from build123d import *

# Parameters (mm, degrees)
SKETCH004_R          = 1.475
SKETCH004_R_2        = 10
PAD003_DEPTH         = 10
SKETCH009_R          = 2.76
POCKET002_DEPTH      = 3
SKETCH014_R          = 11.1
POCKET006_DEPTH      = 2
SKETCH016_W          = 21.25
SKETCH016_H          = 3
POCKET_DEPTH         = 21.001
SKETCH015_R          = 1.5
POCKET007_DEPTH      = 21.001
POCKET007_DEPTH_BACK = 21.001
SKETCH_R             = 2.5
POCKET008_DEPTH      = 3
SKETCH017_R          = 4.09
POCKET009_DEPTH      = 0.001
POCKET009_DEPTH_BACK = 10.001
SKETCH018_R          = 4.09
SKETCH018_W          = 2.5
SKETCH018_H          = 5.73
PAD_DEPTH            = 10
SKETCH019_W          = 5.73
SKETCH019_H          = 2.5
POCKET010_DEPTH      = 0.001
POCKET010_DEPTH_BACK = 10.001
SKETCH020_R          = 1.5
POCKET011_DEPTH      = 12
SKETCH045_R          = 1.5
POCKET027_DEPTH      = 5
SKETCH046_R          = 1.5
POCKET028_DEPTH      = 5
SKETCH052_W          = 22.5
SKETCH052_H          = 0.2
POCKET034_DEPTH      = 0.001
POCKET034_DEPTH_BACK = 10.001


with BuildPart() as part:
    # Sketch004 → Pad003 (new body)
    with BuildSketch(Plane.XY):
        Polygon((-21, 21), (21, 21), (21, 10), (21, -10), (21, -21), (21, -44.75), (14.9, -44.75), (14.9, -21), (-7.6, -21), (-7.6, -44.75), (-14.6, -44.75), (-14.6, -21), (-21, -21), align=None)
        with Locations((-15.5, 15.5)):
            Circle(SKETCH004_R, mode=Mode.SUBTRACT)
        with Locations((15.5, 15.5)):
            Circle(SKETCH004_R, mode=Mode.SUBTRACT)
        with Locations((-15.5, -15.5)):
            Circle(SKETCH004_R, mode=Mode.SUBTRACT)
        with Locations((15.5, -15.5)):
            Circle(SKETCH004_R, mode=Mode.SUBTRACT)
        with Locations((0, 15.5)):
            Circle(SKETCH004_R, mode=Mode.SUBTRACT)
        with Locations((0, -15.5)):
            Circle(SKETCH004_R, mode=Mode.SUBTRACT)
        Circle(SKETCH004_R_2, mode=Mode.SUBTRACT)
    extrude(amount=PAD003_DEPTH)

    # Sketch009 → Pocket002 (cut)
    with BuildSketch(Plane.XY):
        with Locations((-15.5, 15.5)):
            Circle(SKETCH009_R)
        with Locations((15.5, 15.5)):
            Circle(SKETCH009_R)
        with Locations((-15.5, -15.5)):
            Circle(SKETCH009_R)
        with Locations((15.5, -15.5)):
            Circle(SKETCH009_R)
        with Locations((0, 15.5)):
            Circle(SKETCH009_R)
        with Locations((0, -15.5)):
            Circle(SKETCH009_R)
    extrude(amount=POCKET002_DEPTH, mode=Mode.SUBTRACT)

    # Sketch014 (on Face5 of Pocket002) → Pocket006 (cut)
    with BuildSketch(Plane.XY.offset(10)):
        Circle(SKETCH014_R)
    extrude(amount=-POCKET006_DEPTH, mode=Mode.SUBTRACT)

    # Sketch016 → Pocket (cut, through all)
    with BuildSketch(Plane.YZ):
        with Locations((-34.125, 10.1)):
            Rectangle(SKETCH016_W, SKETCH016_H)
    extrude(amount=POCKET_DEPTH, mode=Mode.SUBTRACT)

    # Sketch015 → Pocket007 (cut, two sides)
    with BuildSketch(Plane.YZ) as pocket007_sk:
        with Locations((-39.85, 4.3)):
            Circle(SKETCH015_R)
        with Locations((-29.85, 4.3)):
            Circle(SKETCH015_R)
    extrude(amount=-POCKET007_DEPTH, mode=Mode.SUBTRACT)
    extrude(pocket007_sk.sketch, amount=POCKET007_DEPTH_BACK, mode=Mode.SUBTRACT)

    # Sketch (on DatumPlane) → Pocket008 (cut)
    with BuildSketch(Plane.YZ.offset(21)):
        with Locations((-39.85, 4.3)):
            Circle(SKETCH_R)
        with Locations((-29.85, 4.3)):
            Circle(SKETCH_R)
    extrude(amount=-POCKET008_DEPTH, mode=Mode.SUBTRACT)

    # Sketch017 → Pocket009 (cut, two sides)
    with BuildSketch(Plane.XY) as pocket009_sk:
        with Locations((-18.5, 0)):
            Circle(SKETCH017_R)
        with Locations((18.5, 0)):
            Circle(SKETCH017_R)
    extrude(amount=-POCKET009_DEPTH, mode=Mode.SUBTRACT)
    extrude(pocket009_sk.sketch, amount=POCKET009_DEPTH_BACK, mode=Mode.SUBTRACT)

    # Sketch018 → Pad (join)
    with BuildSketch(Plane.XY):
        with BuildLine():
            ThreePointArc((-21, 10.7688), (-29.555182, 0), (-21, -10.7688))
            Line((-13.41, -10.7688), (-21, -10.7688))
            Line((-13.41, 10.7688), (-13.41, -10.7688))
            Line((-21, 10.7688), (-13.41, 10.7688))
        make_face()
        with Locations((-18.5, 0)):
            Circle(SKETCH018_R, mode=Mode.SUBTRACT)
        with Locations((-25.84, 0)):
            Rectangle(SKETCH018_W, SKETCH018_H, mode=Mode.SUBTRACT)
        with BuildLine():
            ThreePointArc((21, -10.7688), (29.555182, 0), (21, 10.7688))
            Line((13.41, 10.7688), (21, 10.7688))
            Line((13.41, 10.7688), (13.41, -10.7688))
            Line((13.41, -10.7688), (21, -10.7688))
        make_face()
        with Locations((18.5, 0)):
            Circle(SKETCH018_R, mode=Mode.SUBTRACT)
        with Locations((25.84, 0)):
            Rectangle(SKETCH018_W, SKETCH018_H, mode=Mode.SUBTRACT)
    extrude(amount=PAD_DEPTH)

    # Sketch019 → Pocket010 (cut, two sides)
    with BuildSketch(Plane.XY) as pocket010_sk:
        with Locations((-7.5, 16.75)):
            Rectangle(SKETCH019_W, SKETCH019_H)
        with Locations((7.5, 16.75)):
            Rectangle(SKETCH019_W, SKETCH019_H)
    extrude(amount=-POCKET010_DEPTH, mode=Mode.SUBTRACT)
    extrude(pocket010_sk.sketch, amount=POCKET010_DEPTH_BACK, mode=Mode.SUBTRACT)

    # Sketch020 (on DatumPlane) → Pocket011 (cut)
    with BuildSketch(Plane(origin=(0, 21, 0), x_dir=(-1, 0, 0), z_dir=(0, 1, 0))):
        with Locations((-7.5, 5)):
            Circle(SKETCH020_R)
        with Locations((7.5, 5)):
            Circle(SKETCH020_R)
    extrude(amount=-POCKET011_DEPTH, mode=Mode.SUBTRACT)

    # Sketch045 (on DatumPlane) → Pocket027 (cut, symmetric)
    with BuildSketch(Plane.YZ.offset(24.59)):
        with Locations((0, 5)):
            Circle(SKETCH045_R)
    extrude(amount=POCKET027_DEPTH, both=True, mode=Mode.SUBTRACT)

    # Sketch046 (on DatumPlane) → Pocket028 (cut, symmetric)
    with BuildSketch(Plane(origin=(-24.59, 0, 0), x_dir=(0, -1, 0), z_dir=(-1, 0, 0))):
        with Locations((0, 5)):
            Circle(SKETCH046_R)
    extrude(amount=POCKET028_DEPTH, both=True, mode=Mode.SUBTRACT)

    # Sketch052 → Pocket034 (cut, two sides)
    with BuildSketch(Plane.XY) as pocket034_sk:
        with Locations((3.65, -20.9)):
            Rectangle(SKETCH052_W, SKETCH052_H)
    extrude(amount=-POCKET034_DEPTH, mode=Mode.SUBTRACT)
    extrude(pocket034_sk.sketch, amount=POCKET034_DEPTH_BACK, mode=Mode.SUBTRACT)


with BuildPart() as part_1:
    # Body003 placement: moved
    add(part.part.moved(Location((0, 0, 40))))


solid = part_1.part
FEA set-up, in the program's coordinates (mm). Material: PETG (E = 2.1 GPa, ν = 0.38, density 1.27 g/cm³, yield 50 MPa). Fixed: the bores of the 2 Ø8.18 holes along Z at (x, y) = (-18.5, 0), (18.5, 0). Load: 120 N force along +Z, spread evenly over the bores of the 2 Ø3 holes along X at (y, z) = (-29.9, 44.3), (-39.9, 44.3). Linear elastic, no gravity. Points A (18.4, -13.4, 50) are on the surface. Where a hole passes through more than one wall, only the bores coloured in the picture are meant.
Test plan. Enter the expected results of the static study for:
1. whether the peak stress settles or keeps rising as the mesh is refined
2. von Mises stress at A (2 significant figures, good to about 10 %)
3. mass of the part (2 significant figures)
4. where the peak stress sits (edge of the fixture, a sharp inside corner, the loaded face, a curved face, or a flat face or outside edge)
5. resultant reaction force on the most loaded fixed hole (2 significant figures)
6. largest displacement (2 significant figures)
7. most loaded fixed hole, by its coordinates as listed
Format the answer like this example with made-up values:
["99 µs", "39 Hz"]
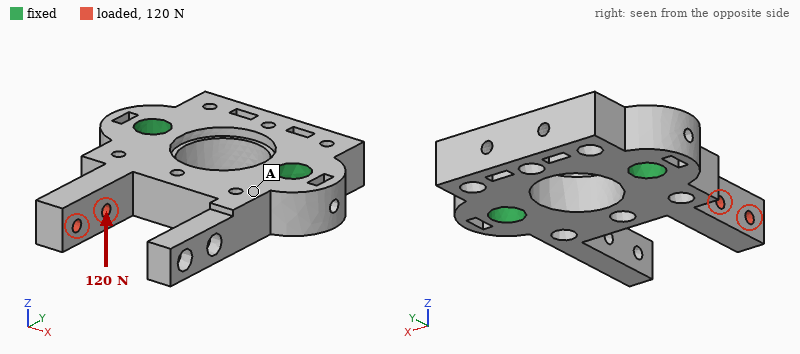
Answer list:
["keeps rising", "2.5 MPa", "22 g", "a sharp inside corner", "95 N", "0.99 mm", "(-18.5, 0)"]
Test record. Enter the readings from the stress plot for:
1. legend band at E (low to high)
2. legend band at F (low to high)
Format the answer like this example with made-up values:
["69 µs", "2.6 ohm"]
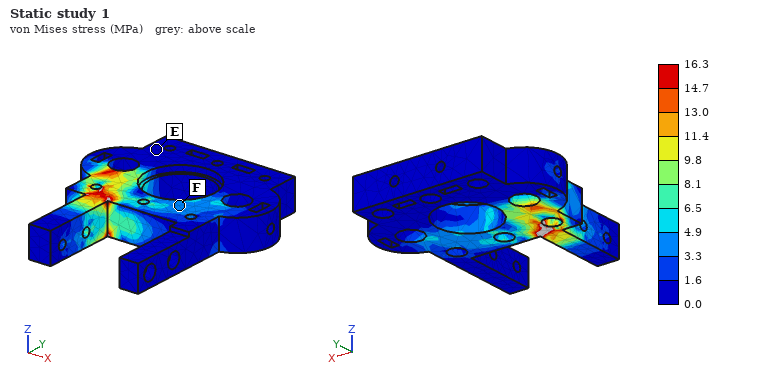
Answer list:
["0.0 to 1.6 MPa", "3.3 to 4.9 MPa"]
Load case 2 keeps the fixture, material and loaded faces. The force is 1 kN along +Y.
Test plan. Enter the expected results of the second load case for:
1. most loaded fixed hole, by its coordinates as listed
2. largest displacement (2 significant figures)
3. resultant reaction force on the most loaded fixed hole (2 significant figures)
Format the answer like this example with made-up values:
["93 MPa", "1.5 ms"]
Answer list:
["(-18.5, 0)", "0.47 mm", "880 N"]
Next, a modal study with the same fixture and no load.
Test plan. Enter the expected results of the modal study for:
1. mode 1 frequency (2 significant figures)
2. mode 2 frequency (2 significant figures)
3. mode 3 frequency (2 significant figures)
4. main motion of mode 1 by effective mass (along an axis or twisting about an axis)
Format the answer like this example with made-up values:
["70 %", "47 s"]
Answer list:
["1500 Hz", "1600 Hz", "1700 Hz", "along Z"]
